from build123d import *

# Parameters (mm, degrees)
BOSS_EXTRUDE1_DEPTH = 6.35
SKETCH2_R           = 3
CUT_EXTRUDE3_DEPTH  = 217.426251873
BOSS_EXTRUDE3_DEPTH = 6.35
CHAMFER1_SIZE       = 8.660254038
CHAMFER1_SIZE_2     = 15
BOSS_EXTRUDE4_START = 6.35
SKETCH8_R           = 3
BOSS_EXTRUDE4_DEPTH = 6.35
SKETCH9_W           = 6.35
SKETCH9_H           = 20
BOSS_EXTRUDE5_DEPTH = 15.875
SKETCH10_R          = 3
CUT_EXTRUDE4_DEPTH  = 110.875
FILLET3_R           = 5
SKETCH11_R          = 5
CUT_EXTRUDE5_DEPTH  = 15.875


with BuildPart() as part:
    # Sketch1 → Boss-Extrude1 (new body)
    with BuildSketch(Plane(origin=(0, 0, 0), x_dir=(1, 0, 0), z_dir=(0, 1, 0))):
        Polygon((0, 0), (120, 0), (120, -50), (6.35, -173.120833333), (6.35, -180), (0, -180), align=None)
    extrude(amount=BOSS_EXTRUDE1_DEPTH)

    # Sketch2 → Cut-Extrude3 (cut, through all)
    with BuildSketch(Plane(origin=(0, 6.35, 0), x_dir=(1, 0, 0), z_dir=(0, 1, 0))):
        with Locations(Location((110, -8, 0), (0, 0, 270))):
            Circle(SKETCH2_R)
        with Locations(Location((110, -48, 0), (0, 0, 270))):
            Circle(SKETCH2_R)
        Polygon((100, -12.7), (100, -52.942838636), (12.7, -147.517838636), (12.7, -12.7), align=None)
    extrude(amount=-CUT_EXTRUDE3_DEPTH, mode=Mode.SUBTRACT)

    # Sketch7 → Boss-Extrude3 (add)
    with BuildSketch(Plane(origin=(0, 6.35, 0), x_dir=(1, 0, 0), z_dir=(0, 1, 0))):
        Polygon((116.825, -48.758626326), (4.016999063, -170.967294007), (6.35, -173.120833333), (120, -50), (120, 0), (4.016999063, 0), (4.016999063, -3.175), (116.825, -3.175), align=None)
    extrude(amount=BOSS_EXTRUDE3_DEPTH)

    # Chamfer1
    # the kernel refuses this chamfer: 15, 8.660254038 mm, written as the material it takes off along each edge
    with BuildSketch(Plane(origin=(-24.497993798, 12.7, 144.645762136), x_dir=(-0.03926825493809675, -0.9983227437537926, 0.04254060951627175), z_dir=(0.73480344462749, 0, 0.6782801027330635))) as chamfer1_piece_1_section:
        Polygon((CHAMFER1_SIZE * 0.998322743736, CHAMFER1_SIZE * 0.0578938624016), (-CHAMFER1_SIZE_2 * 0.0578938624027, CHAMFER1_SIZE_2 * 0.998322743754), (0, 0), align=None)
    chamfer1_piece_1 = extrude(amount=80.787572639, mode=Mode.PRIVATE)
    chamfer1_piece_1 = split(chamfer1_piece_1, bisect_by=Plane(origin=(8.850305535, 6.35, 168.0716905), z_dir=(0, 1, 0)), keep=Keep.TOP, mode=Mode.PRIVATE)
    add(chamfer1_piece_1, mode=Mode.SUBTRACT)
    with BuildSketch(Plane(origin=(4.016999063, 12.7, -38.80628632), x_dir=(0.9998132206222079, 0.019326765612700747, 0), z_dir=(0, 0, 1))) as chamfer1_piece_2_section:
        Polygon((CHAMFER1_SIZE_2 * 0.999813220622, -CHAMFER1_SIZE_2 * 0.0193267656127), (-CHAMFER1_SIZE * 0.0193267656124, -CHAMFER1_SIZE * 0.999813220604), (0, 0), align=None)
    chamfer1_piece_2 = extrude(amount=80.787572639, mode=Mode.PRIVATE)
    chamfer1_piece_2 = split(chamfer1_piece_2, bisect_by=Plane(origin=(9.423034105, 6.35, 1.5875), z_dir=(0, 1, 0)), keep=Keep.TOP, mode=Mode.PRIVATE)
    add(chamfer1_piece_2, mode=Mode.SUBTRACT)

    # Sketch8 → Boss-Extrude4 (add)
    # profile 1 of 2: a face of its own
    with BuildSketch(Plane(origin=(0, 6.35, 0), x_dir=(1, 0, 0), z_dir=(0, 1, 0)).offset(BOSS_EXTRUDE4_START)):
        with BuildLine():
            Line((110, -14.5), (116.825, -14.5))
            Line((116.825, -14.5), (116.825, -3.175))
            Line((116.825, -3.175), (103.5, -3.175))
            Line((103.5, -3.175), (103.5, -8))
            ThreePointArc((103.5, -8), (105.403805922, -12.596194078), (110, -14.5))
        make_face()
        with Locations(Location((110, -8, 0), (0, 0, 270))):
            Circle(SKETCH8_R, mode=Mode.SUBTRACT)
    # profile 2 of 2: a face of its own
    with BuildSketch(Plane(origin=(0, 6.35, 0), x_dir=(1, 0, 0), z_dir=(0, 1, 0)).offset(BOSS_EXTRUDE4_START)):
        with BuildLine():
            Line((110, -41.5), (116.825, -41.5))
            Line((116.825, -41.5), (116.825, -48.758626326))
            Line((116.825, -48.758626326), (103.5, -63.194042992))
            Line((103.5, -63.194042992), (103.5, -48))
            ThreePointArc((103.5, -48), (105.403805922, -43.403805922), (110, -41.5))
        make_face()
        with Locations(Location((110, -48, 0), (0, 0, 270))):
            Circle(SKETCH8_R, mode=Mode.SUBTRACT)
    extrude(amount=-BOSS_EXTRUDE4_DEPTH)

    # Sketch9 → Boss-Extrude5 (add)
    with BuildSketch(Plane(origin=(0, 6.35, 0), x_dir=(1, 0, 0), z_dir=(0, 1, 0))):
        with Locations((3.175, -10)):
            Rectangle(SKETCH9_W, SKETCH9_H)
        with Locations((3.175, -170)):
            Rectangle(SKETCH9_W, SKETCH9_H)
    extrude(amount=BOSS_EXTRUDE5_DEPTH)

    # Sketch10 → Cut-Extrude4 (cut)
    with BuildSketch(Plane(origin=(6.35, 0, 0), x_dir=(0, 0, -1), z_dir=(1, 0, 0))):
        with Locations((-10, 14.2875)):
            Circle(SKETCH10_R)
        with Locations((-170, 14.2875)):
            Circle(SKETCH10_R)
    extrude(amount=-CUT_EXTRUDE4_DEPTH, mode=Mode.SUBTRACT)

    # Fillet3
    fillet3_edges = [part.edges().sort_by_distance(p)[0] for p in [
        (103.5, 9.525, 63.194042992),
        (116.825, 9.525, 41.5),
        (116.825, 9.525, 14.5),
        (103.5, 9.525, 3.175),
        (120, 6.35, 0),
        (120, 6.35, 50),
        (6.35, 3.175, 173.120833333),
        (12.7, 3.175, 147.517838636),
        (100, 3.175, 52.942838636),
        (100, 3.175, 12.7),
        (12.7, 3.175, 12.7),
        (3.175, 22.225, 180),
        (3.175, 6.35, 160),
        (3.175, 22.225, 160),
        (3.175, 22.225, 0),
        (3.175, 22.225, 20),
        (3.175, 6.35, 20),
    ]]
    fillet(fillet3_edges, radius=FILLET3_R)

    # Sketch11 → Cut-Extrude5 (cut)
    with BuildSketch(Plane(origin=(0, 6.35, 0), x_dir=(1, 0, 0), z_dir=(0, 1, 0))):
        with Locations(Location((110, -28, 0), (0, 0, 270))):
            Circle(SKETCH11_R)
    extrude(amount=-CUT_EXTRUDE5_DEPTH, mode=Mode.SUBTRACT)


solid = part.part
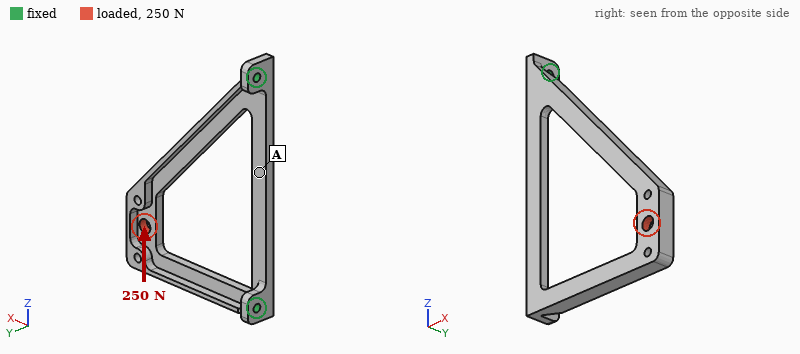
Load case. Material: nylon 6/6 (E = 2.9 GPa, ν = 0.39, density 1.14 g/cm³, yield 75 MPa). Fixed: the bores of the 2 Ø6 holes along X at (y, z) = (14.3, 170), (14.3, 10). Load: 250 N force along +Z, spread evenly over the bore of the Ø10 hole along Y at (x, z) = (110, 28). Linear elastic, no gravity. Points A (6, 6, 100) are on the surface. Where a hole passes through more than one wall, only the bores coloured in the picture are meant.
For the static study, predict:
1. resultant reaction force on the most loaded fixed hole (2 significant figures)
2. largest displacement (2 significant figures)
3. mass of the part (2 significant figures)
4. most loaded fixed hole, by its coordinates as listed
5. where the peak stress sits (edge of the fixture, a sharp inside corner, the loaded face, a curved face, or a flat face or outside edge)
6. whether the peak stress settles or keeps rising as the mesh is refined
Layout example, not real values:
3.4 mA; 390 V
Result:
230 N; 1.6 mm; 57 g; (14.3, 170); edge of the fixture; keeps rising
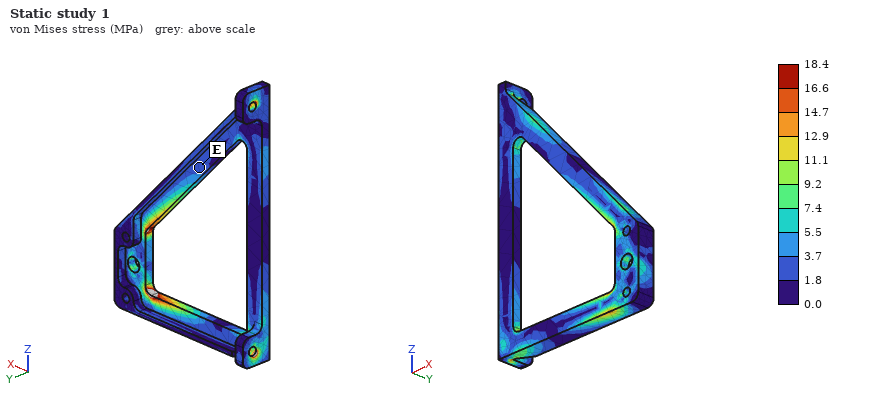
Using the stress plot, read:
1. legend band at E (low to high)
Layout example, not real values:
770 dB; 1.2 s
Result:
1.8 to 3.7 MPa
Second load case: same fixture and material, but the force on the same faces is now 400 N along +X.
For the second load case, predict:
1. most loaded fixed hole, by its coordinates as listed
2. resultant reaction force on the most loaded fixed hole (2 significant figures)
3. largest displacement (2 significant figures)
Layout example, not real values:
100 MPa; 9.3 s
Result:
(14.3, 10); 340 N; 2.1 mm
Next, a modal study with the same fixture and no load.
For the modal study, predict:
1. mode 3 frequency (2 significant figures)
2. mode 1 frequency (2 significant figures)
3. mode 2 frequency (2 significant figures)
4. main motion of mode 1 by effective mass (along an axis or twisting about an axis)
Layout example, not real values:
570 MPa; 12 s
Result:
400 Hz; 86 Hz; 290 Hz; along Y
